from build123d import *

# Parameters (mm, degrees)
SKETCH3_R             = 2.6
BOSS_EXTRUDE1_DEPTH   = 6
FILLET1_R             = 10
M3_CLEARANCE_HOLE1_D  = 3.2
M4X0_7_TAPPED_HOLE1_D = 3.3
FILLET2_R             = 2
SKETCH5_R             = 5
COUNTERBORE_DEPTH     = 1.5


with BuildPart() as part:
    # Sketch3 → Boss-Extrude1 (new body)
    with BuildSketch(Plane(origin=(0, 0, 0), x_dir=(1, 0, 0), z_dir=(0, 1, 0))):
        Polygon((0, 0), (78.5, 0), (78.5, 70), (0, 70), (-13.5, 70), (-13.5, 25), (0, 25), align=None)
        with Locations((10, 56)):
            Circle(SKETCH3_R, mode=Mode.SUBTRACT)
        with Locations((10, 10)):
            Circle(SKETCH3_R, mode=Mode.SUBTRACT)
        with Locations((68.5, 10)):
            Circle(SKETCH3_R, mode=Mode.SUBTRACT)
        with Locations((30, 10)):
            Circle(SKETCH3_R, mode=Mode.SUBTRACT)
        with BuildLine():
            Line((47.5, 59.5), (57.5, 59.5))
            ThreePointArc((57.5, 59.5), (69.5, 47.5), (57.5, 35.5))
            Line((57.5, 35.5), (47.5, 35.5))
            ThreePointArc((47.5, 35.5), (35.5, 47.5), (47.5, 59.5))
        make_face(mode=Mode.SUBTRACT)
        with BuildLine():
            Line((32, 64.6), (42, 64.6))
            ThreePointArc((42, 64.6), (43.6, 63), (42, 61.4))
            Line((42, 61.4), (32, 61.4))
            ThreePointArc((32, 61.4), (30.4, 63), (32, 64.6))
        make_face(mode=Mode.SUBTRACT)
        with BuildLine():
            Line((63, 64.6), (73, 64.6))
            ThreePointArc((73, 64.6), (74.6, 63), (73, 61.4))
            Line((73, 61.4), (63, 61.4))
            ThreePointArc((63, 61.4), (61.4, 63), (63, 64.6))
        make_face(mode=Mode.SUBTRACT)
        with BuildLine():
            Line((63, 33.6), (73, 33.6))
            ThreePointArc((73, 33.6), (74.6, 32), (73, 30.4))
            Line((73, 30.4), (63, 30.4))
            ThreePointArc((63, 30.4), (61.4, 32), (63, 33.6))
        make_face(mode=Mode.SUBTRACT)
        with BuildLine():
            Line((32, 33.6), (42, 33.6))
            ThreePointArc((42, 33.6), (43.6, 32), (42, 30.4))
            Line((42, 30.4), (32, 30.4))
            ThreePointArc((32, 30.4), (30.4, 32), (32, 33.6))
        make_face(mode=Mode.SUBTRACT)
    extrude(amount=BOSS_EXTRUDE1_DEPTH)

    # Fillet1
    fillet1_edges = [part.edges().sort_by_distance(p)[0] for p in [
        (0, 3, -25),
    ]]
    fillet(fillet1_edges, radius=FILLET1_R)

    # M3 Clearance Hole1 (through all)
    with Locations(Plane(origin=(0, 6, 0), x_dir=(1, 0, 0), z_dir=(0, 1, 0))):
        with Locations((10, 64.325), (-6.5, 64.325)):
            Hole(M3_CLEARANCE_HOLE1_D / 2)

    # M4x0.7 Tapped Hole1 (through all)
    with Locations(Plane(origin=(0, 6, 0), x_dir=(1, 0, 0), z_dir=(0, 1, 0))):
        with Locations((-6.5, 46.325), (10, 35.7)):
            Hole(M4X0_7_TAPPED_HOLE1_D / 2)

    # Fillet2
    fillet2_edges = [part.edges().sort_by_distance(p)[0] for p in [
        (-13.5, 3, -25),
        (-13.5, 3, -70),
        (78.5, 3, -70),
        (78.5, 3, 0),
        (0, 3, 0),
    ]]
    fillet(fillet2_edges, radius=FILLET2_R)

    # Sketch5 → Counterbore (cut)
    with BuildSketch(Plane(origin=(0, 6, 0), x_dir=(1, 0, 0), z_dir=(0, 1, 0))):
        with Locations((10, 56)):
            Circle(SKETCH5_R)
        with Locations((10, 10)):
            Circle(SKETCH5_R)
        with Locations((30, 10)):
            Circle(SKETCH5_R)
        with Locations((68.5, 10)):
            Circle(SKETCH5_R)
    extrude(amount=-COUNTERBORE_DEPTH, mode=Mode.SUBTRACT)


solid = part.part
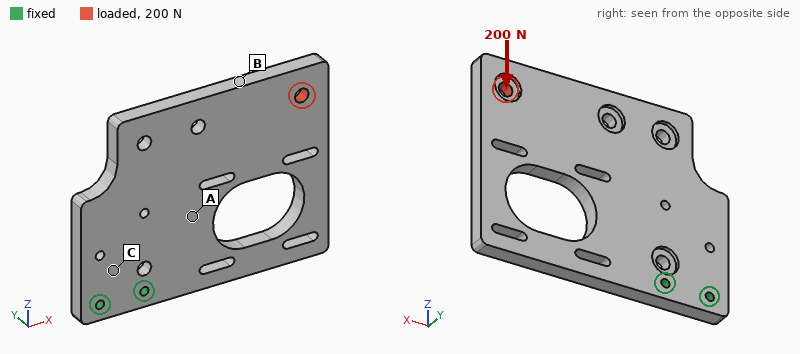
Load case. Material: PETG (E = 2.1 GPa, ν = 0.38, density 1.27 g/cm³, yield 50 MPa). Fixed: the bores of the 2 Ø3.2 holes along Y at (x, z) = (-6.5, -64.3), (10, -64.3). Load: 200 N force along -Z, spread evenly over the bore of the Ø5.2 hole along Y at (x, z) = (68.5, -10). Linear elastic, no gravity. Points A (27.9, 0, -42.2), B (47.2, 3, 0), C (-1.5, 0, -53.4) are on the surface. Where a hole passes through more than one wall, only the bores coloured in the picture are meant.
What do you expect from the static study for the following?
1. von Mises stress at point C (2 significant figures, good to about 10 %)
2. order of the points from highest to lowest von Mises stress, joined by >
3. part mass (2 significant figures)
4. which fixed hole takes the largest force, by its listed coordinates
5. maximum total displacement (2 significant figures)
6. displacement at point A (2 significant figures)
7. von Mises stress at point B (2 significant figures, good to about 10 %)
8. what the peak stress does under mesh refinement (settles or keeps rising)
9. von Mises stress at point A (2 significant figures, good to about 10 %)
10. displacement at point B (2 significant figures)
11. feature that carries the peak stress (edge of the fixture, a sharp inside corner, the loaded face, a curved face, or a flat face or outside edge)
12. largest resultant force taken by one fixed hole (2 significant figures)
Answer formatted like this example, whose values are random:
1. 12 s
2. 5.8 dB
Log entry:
1. 6.5 MPa
2. C > A > B
3. 39 g
4. (10, -64.3)
5. 1.3 mm
6. 0.35 mm
7. 1.9 MPa
8. keeps rising
9. 3.3 MPa
10. 0.96 mm
11. edge of the fixture
12. 800 N
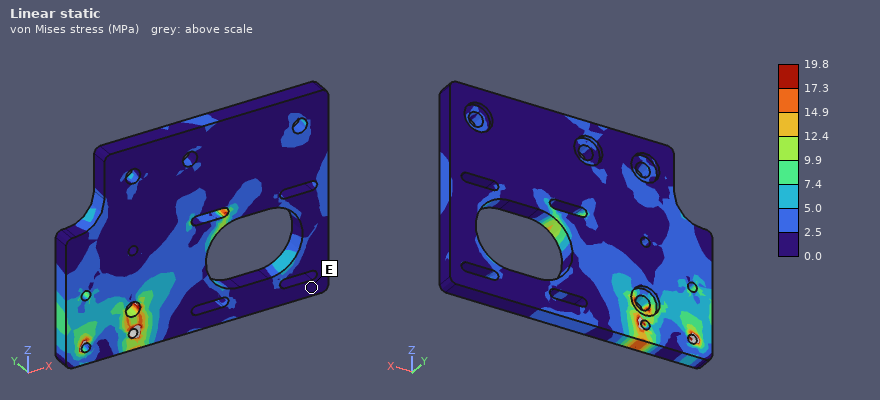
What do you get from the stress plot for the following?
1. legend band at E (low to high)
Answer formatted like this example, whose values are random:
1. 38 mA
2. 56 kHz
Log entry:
1. 0.0 to 2.5 MPa
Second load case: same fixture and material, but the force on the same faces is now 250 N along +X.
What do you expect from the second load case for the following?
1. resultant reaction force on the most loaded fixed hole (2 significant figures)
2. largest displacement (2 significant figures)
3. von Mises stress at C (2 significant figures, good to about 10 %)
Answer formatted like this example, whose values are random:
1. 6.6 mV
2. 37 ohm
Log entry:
1. 730 N
2. 1.3 mm
3. 8.7 MPa
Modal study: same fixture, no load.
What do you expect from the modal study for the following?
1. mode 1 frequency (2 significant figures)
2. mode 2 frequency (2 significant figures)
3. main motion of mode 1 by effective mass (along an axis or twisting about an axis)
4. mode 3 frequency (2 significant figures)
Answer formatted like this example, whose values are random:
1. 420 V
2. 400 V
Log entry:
1. 140 Hz
2. 300 Hz
3. along Y
4. 520 Hz
